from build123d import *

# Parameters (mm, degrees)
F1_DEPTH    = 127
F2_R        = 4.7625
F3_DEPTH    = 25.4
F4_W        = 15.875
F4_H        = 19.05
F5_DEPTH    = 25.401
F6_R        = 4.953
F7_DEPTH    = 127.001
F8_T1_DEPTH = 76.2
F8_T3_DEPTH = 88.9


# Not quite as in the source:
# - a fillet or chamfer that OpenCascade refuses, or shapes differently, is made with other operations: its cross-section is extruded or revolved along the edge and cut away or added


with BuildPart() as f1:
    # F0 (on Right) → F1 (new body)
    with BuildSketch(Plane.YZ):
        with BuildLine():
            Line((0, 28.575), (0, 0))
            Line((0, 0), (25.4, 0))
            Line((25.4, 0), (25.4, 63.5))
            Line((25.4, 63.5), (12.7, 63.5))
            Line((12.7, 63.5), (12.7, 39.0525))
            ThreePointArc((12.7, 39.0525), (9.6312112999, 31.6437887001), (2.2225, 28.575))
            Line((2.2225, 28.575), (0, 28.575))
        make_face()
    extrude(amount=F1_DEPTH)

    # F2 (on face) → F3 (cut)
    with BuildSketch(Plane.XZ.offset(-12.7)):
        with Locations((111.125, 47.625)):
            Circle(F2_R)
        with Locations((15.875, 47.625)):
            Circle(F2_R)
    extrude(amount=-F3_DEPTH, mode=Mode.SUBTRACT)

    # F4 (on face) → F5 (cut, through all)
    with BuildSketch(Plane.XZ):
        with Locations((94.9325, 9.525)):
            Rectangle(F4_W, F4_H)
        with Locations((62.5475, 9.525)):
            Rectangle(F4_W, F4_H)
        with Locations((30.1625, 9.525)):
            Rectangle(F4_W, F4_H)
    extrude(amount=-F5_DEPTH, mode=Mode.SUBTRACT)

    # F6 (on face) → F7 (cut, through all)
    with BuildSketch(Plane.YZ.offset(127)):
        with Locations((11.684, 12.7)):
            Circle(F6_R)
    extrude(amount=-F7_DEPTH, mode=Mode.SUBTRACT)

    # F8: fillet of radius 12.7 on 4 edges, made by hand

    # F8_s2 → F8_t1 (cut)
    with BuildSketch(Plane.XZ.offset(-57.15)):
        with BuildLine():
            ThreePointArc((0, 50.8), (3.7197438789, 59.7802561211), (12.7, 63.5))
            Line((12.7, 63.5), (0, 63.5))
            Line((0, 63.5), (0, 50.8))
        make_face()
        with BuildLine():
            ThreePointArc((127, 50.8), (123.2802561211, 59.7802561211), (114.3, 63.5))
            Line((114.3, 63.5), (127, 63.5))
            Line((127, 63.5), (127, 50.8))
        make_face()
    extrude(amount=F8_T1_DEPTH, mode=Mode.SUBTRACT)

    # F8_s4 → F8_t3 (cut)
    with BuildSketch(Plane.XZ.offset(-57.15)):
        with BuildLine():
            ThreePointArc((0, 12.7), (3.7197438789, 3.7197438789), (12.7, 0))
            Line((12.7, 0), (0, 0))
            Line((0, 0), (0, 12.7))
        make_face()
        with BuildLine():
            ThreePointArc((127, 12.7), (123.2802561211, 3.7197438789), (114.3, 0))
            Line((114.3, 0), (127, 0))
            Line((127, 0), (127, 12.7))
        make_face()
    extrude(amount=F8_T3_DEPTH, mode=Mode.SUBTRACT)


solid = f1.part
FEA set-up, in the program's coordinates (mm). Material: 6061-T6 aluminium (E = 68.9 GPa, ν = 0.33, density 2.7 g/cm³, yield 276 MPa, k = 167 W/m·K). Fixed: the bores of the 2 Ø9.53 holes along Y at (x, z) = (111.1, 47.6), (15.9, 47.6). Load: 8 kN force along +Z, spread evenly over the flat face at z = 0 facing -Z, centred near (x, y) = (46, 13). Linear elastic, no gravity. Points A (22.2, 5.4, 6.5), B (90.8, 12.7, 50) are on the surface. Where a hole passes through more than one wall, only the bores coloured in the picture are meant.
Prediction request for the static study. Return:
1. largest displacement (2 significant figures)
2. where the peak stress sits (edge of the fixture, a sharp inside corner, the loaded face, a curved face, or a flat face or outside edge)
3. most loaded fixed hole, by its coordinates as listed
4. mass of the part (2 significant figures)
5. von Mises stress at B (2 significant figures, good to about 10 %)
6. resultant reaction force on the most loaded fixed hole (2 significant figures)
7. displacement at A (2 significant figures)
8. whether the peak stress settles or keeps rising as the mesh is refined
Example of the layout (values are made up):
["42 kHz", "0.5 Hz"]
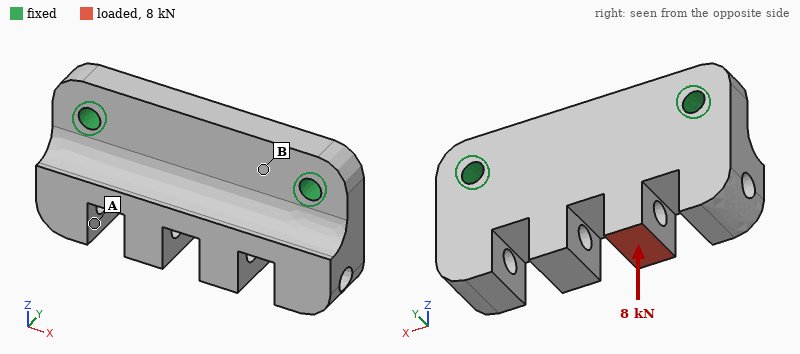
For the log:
["85 µm", "edge of the fixture", "(15.9, 47.6)", "320 g", "19 MPa", "5.9 kN", "39 µm", "keeps rising"]
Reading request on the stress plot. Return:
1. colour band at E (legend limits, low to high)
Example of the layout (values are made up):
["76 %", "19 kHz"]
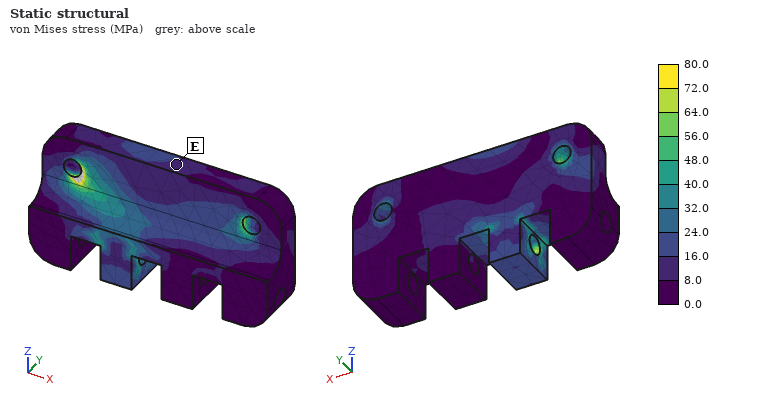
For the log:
["8.0 to 16.0 MPa"]
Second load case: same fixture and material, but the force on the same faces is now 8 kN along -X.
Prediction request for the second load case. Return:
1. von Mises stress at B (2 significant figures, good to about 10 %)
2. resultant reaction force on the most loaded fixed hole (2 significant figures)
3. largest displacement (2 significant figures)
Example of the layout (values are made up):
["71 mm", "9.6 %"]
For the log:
["15 MPa", "5.9 kN", "0.15 mm"]
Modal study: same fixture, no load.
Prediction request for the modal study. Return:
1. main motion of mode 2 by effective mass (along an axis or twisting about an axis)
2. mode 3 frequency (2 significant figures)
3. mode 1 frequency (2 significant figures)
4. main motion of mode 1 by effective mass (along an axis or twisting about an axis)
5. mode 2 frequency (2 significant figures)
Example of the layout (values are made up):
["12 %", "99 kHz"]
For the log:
["twisting about Z", "6300 Hz", "3100 Hz", "along Y", "4800 Hz"]
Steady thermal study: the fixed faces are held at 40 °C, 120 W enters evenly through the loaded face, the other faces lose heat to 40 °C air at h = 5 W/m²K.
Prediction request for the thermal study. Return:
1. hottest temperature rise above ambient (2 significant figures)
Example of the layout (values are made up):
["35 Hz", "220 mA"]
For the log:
["82 K"]
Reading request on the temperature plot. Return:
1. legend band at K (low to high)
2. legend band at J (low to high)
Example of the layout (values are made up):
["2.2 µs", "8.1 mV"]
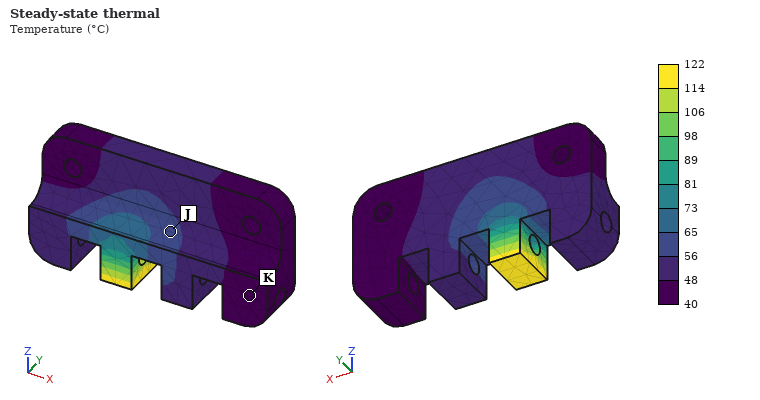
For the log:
["40 to 48 °C", "56 to 65 °C"]
